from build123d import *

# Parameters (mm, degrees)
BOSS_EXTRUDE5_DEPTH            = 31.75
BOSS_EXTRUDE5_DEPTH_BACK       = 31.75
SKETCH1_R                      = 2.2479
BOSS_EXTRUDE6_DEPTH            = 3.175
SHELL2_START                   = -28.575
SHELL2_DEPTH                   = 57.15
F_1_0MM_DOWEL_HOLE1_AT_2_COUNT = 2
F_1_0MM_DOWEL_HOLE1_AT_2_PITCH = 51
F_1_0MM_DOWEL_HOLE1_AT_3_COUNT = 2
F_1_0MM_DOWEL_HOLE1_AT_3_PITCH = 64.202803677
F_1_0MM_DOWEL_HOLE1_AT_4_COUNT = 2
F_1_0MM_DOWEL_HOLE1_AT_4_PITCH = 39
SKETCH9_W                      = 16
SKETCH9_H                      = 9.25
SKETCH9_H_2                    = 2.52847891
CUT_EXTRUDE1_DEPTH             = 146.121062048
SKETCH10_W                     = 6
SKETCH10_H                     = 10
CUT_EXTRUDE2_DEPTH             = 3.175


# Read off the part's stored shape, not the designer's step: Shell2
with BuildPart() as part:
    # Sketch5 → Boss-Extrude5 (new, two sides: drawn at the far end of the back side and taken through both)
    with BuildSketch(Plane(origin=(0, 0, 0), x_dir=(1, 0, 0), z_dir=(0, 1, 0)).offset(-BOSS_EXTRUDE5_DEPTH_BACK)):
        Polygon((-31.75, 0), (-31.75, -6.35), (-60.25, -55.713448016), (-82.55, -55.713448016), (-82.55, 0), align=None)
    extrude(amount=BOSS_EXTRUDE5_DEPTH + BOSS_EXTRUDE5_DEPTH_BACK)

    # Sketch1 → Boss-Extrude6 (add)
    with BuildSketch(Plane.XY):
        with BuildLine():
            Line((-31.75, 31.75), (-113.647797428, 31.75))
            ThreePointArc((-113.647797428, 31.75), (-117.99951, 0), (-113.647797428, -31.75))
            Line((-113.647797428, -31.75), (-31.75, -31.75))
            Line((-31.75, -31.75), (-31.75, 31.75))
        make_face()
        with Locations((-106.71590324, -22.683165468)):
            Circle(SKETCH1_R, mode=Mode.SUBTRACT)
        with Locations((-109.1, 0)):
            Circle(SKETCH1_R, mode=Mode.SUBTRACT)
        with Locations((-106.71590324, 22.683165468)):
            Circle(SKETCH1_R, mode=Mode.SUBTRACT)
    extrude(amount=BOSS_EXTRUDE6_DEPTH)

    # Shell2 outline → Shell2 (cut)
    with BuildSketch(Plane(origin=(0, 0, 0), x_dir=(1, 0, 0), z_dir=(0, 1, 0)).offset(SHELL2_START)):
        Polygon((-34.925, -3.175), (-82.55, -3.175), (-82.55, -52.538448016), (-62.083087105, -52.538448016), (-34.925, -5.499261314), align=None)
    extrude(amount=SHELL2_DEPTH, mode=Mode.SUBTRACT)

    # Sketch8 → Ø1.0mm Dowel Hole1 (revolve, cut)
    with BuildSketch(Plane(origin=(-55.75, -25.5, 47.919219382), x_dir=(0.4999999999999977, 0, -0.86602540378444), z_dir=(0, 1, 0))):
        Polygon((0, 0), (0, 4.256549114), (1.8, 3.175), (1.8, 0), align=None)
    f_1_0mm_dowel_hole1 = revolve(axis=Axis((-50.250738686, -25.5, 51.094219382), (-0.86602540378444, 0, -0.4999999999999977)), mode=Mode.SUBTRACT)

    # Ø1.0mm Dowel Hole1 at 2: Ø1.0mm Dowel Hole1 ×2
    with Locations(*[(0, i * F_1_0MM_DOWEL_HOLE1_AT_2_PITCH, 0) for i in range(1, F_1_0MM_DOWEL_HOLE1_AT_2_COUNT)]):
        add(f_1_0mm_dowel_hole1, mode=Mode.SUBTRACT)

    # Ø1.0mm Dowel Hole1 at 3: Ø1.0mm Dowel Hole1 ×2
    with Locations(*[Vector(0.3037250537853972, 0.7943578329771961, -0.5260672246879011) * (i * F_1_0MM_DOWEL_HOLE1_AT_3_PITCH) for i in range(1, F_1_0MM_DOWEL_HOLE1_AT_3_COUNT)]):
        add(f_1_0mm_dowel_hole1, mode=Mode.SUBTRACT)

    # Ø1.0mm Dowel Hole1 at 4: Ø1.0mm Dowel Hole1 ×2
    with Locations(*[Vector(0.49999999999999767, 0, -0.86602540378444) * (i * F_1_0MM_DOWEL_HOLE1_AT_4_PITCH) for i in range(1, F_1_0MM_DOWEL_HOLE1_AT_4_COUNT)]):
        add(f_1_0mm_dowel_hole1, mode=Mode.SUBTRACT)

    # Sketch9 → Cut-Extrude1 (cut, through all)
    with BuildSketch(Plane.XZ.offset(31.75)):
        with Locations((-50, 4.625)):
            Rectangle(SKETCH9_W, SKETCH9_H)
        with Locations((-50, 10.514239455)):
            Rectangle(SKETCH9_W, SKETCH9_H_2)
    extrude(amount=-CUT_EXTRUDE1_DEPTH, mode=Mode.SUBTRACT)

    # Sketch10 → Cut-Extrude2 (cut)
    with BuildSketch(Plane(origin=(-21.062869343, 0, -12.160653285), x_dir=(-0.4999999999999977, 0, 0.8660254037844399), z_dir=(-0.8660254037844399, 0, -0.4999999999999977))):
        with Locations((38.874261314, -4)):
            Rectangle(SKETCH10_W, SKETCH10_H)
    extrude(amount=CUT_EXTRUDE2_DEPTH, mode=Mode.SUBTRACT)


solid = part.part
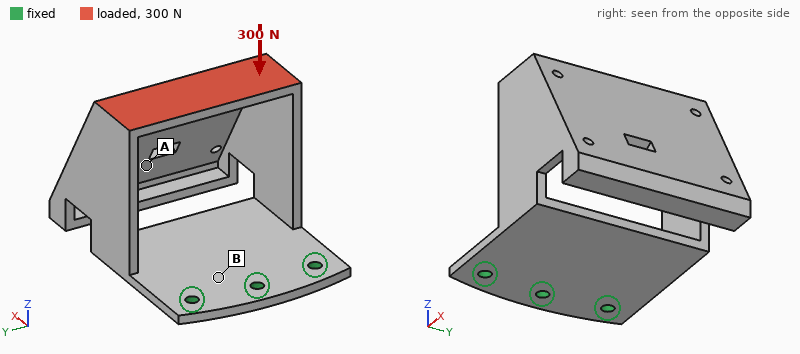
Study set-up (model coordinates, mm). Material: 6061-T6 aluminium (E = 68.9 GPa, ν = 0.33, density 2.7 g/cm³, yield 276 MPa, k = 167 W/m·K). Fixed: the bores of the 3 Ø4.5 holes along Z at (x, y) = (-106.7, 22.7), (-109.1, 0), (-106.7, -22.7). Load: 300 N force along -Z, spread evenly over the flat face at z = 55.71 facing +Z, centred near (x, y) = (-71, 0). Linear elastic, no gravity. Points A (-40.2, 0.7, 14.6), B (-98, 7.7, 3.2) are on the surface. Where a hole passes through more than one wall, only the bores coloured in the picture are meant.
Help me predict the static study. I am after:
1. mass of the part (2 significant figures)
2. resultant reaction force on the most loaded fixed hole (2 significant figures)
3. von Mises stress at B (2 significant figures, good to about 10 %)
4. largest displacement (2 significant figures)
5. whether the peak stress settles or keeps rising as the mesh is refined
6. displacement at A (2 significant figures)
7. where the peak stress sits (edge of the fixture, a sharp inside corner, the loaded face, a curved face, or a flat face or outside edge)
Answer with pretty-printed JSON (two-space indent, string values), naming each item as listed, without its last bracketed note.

{
  "mass of the part": "110 g",
  "resultant reaction force on the most loaded fixed hole": "140 N",
  "von Mises stress at B": "59 MPa",
  "largest displacement": "1.00 mm",
  "whether the peak stress settles or keeps rising as the mesh is refined": "keeps rising",
  "displacement at A": "0.88 mm",
  "where the peak stress sits": "edge of the fixture"
}
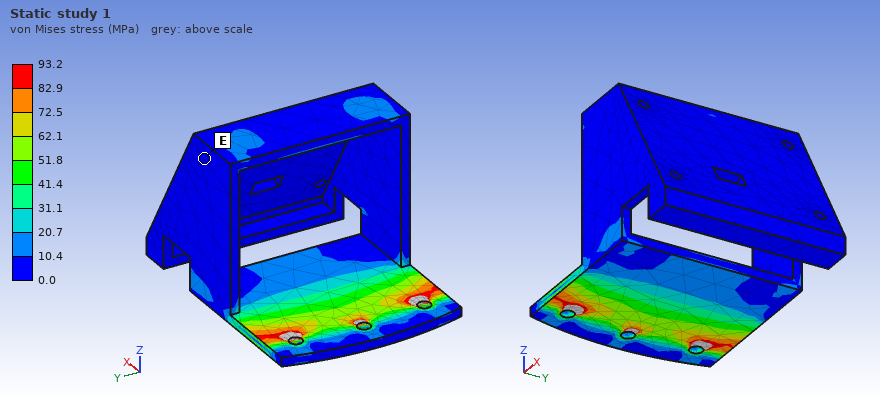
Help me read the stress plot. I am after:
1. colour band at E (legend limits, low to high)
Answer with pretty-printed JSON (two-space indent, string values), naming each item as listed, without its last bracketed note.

{
  "colour band at E": "0.0 to 10.4 MPa"
}
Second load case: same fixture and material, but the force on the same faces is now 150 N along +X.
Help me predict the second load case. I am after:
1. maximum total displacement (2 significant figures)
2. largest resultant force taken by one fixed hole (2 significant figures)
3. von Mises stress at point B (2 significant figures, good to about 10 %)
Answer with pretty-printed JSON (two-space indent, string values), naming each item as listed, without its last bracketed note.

{
  "maximum total displacement": "1.4 mm",
  "largest resultant force taken by one fixed hole": "70 N",
  "von Mises stress at point B": "66 MPa"
}
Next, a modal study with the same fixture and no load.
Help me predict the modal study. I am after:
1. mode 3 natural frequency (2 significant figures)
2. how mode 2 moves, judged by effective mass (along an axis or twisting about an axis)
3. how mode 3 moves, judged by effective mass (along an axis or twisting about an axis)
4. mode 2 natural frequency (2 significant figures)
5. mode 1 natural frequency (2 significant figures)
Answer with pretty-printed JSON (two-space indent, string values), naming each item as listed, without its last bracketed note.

{
  "mode 3 natural frequency": "1100 Hz",
  "how mode 2 moves, judged by effective mass": "along Y",
  "how mode 3 moves, judged by effective mass": "along Y",
  "mode 2 natural frequency": "480 Hz",
  "mode 1 natural frequency": "220 Hz"
}
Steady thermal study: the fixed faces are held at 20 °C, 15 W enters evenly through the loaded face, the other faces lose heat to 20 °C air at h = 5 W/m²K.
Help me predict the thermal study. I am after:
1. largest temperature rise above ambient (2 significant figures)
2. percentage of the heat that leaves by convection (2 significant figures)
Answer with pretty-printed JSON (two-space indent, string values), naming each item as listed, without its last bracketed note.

{
  "largest temperature rise above ambient": "38 K",
  "percentage of the heat that leaves by convection": "18 %"
}
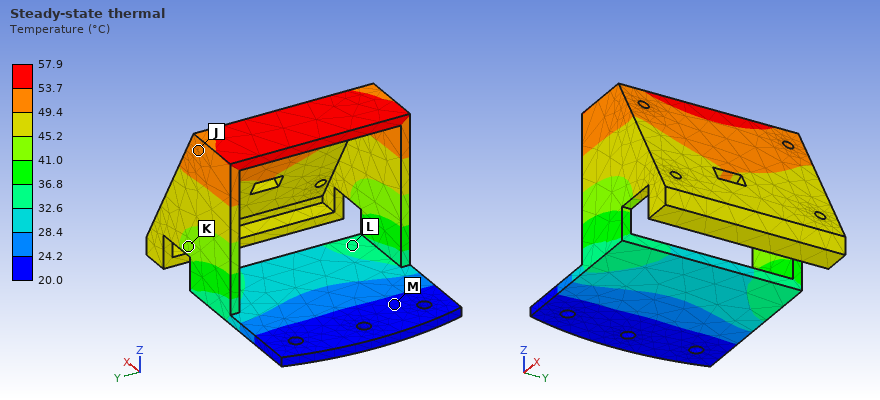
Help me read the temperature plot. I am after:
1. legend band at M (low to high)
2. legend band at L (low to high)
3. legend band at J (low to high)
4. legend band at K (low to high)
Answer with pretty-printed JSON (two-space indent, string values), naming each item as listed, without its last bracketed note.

{
  "legend band at M": "20.0 to 24.2 °C",
  "legend band at L": "32.6 to 36.8 °C",
  "legend band at J": "49.4 to 53.7 °C",
  "legend band at K": "41.0 to 45.2 °C"
}
